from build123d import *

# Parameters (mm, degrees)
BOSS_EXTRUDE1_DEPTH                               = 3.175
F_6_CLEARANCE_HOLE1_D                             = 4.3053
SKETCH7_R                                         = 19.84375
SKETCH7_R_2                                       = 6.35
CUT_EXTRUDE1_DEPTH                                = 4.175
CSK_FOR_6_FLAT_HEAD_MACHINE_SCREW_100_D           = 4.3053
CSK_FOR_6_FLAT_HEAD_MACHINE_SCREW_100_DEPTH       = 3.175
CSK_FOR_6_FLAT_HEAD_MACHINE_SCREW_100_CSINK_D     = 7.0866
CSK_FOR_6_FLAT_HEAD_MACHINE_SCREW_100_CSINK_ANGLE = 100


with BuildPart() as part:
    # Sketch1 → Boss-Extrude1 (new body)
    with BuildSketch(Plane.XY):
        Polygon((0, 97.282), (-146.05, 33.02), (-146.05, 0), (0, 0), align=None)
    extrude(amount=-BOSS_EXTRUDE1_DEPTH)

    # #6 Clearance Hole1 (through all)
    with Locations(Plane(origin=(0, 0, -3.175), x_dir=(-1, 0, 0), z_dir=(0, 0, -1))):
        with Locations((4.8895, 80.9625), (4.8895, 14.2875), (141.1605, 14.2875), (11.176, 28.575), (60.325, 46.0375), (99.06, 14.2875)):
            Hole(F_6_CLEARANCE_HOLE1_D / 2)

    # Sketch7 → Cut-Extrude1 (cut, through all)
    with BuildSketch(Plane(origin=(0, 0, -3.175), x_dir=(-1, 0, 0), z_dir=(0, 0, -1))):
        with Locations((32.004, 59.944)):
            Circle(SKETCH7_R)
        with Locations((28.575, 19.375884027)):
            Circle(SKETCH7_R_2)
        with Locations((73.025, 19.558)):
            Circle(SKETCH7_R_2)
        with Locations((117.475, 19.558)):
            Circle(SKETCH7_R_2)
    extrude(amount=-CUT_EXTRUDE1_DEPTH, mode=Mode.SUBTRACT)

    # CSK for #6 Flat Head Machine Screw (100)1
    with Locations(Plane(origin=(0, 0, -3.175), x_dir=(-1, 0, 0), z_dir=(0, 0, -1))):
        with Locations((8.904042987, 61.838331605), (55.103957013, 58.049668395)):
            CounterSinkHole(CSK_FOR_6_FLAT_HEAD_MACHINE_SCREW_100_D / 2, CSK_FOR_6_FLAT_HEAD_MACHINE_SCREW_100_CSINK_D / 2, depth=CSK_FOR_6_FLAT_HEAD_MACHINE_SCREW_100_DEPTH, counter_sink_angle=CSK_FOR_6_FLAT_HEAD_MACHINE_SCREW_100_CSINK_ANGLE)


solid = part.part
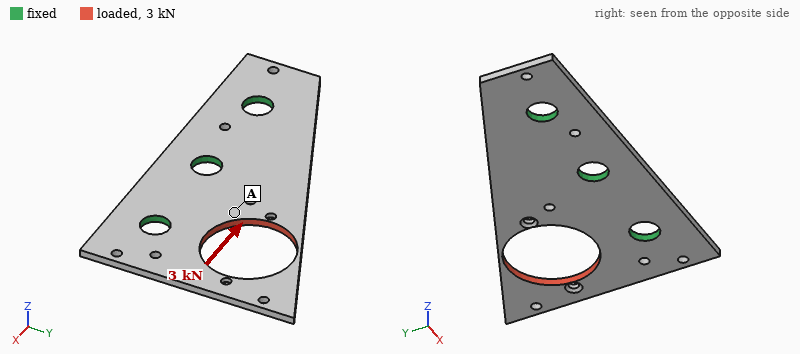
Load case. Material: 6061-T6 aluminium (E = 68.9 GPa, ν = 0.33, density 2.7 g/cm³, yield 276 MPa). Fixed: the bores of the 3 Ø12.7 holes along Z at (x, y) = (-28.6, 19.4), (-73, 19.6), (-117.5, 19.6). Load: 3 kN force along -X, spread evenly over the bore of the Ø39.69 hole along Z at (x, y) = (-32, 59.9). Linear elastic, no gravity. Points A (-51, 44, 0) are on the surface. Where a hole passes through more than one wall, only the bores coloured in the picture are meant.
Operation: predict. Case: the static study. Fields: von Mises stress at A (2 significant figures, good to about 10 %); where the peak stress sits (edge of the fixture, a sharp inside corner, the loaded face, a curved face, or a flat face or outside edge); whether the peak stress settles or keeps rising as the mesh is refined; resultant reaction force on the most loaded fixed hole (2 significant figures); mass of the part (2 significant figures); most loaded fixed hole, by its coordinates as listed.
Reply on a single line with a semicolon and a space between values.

23 MPa; a sharp inside corner; keeps rising; 2.0 kN; 67 g; (-28.6, 19.4)
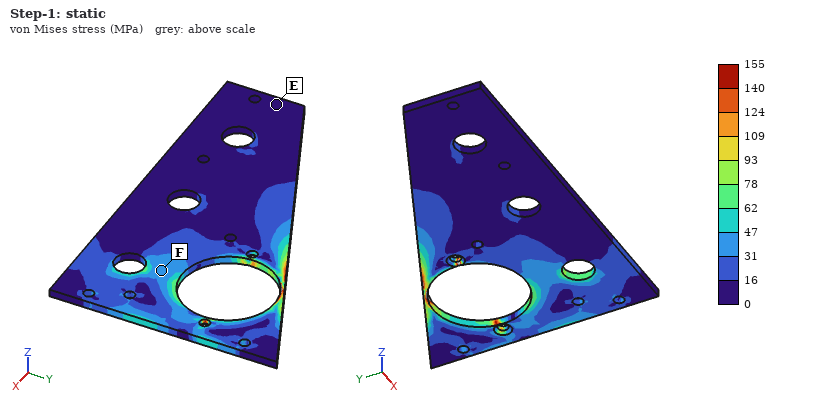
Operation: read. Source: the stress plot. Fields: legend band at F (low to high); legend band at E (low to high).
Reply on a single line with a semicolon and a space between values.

31 to 47 MPa; 0 to 16 MPa
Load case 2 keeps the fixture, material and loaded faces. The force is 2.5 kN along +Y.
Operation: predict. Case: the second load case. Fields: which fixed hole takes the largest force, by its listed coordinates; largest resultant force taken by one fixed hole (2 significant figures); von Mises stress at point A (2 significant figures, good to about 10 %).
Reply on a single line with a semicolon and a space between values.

(-28.6, 19.4); 2.0 kN; 15 MPa
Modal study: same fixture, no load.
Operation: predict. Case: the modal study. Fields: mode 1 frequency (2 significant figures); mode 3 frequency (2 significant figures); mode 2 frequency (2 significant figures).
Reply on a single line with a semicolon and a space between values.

620 Hz; 2600 Hz; 1700 Hz
